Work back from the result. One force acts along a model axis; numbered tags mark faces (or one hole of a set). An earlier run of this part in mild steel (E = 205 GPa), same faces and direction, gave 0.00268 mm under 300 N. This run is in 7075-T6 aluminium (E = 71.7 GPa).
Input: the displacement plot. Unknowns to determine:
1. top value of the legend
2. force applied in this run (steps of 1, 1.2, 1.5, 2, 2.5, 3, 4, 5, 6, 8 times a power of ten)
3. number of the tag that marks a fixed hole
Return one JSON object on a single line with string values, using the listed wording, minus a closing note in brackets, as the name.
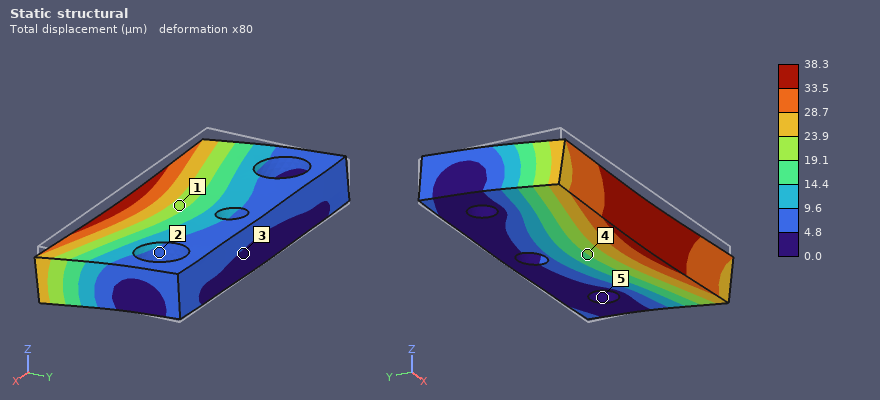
{"top value of the legend": "38.3 µm", "force applied in this run": "1.5 kN", "number of the tag that marks a fixed hole": "5"}
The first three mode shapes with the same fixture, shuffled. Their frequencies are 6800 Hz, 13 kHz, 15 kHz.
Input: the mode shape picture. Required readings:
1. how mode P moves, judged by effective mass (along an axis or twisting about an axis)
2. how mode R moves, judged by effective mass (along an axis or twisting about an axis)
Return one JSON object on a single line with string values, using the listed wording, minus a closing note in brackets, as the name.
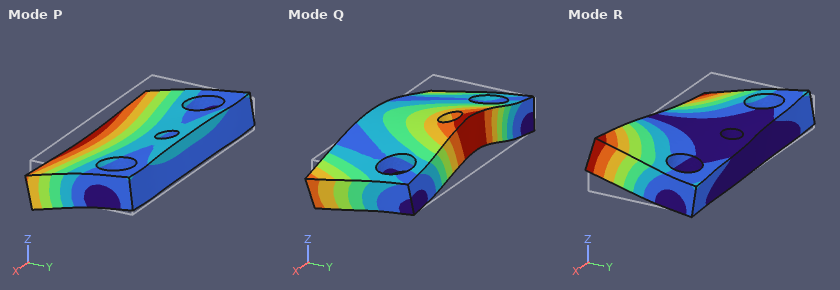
{"how mode P moves, judged by effective mass": "along Z", "how mode R moves, judged by effective mass": "twisting about Y"}
